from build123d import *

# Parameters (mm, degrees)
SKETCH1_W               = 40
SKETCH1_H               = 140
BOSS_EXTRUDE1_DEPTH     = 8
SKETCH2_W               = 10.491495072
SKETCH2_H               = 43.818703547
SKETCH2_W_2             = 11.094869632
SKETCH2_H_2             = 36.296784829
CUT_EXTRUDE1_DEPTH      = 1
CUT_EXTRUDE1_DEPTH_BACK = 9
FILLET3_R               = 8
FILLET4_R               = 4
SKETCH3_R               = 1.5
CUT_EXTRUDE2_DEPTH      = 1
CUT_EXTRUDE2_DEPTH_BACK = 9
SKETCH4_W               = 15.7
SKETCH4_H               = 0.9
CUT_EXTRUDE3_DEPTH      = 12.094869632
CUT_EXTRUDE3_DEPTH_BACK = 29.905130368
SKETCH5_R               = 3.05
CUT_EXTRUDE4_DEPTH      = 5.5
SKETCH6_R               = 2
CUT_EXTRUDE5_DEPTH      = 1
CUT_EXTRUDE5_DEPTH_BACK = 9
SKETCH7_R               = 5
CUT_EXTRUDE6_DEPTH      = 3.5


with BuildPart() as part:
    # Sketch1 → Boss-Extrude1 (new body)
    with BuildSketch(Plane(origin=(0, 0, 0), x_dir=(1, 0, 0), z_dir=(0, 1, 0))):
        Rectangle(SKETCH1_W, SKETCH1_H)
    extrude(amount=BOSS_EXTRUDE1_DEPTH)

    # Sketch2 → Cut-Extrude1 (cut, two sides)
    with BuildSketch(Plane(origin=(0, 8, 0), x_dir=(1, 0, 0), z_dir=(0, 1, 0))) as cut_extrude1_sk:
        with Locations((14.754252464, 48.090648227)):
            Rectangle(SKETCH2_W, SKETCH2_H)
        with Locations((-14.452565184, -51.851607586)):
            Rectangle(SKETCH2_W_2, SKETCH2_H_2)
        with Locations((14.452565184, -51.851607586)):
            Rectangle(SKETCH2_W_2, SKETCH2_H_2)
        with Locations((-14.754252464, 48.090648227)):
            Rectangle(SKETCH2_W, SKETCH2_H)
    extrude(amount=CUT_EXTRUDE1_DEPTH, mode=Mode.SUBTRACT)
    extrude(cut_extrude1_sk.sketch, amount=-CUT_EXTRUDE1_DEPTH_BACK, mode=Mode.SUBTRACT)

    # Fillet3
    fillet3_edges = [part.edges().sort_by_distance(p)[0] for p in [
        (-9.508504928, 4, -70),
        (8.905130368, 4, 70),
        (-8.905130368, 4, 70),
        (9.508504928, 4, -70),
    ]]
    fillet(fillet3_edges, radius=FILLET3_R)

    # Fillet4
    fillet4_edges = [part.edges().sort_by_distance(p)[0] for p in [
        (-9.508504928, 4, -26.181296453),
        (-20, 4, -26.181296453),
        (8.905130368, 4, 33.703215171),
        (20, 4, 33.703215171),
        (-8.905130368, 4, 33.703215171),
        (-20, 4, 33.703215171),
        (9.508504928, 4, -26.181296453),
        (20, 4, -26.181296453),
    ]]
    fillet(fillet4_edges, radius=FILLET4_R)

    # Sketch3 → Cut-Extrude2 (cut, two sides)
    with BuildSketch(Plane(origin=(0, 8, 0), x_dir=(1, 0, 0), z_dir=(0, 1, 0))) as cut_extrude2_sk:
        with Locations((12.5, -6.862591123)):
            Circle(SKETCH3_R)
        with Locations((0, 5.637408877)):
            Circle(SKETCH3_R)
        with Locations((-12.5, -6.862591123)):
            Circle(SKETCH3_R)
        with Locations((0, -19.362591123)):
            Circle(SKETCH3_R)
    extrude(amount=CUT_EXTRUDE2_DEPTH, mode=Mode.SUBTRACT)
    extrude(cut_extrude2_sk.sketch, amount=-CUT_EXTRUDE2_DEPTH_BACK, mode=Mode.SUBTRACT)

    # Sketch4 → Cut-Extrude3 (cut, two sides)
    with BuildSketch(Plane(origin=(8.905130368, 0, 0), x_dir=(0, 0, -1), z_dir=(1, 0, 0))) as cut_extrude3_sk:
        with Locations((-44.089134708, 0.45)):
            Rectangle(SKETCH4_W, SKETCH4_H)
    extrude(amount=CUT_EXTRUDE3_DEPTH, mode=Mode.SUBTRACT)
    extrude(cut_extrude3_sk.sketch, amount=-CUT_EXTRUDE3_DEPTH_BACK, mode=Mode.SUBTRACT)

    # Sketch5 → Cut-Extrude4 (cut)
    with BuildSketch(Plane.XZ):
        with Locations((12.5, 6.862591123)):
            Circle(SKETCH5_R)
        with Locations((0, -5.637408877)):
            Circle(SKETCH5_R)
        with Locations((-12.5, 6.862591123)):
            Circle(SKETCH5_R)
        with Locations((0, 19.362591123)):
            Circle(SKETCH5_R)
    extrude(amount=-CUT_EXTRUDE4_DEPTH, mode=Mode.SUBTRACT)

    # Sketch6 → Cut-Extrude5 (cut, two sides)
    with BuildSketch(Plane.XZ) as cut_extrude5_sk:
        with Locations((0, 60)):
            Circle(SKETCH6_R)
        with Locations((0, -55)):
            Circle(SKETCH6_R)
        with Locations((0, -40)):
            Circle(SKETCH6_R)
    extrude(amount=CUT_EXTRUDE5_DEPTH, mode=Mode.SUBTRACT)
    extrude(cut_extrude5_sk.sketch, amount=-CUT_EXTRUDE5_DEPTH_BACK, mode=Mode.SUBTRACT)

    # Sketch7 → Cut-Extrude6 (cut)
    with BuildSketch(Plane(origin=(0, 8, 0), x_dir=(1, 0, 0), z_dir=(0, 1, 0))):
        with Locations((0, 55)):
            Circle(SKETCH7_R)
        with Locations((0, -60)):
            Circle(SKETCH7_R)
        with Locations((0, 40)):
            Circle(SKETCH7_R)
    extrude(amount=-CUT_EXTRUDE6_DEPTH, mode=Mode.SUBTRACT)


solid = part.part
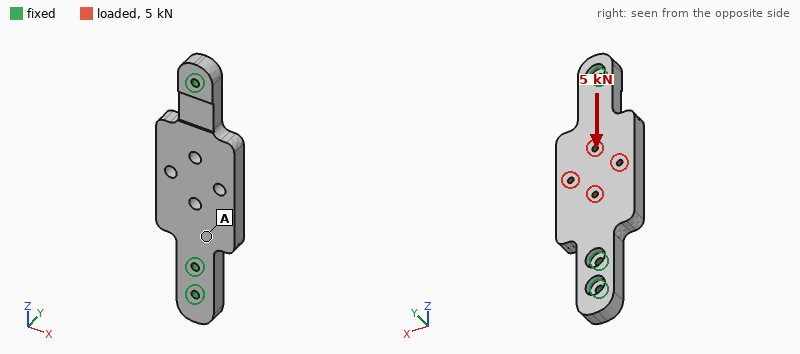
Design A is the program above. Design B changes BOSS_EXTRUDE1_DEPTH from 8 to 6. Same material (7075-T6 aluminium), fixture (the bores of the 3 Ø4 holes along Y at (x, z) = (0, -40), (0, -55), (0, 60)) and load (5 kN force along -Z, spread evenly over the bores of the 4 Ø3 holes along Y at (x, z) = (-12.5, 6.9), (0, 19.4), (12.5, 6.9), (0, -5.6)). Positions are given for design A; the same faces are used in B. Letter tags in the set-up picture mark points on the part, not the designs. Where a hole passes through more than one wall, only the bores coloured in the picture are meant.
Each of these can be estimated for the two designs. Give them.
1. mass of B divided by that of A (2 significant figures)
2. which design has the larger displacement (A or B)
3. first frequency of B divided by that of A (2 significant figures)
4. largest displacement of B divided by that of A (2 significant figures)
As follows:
0.75
B
0.82
2.2
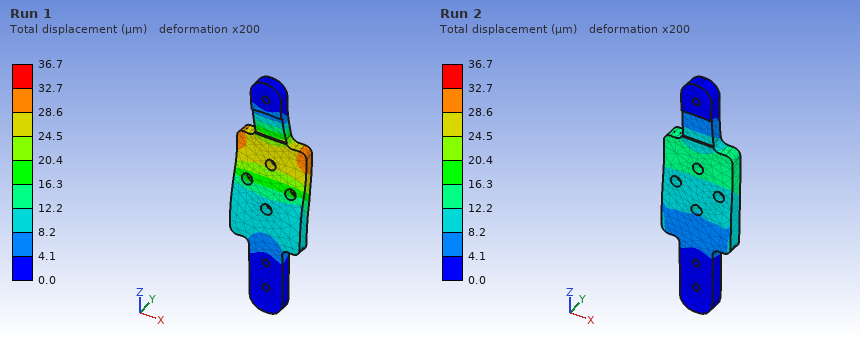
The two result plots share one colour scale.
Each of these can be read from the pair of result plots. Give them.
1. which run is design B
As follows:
Run 1
